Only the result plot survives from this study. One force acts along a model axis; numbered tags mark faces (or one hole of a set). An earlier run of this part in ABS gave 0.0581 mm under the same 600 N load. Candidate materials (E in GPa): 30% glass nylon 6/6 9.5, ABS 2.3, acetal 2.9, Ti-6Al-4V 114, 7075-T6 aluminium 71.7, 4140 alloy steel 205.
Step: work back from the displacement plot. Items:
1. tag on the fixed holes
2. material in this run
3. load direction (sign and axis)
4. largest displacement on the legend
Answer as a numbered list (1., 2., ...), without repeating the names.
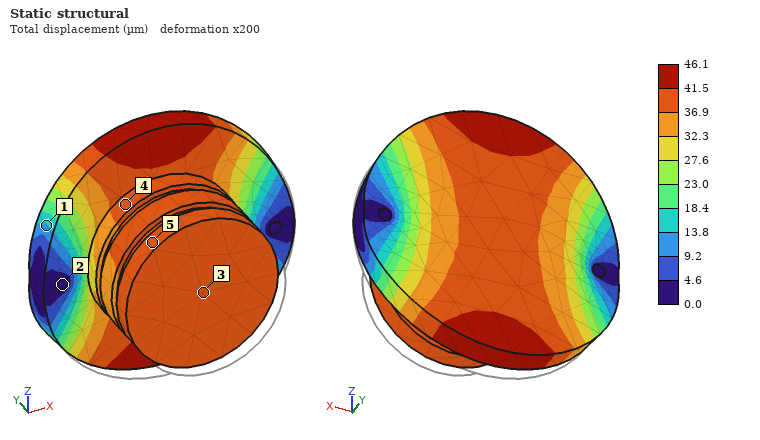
1. 2
2. acetal
3. +Y
4. 46.1 µm
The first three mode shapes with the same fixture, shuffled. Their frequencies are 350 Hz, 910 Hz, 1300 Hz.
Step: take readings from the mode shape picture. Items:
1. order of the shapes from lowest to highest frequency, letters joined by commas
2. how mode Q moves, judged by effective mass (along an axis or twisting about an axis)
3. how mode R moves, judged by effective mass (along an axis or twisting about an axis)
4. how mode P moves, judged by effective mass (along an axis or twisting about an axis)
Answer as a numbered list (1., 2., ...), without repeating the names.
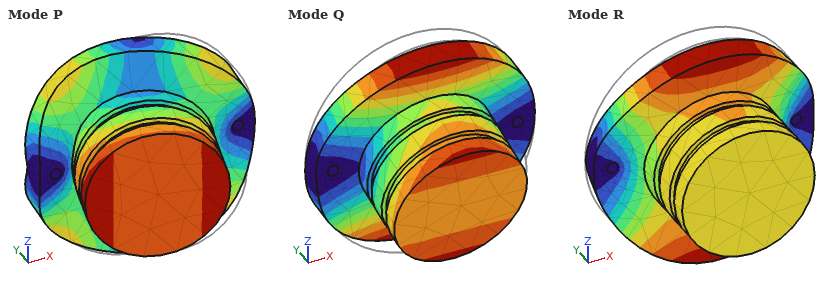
1. Q, R, P
2. along Z
3. along Y
4. along X
